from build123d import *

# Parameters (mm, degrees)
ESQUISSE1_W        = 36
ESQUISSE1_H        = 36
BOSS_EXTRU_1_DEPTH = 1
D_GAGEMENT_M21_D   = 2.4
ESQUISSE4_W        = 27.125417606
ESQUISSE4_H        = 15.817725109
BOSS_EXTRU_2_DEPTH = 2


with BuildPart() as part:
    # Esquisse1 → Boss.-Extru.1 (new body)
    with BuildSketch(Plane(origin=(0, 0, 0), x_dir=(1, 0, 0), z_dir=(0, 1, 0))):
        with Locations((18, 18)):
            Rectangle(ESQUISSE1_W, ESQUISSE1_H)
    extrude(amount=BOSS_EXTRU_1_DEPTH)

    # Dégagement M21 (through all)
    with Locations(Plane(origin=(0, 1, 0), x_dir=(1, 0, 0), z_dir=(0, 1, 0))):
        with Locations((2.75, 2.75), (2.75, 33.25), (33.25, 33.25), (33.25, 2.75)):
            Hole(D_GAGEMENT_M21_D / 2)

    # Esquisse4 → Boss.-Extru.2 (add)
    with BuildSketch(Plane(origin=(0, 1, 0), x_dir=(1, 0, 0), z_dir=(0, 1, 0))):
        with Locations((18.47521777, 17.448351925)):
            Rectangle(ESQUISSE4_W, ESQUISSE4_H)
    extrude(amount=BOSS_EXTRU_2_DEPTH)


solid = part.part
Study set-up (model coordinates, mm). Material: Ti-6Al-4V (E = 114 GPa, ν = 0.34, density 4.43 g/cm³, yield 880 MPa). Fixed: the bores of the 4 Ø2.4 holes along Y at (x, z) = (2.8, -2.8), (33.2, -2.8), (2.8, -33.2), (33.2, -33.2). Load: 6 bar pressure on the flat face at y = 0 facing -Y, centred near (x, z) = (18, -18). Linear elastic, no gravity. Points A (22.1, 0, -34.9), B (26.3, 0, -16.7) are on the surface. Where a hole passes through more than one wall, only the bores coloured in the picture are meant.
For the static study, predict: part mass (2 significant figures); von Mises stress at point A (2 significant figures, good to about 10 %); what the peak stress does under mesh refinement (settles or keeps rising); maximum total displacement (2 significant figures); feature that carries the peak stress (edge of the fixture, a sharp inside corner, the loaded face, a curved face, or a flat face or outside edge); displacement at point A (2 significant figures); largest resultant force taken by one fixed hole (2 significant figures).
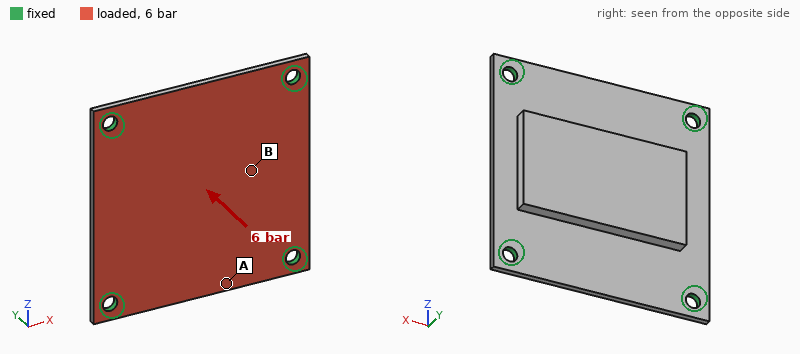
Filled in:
9.5 g
92 MPa
keeps rising
0.10 mm
edge of the fixture
0.087 mm
230 N
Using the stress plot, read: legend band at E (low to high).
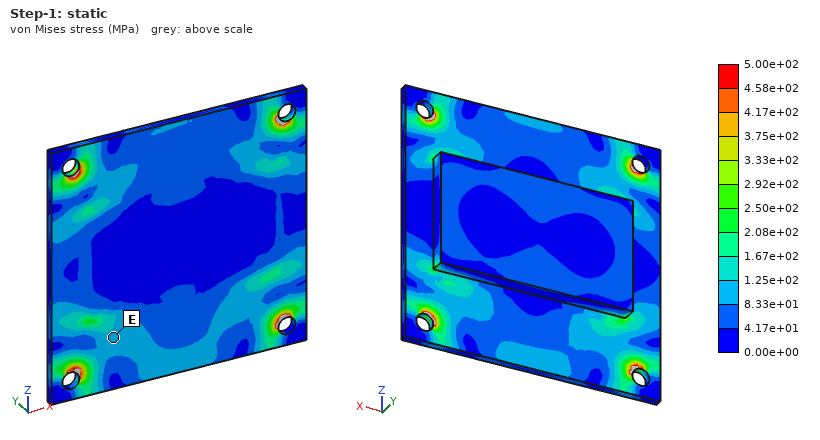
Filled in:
8.33e+01 to 1.25e+02 MPa
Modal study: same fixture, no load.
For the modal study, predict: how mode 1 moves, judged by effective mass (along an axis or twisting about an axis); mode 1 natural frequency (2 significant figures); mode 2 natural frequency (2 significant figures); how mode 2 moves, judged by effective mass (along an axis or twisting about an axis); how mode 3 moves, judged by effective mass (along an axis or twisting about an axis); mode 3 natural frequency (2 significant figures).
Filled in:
along Y
4700 Hz
7700 Hz
twisting about Z
twisting about X
8200 Hz
